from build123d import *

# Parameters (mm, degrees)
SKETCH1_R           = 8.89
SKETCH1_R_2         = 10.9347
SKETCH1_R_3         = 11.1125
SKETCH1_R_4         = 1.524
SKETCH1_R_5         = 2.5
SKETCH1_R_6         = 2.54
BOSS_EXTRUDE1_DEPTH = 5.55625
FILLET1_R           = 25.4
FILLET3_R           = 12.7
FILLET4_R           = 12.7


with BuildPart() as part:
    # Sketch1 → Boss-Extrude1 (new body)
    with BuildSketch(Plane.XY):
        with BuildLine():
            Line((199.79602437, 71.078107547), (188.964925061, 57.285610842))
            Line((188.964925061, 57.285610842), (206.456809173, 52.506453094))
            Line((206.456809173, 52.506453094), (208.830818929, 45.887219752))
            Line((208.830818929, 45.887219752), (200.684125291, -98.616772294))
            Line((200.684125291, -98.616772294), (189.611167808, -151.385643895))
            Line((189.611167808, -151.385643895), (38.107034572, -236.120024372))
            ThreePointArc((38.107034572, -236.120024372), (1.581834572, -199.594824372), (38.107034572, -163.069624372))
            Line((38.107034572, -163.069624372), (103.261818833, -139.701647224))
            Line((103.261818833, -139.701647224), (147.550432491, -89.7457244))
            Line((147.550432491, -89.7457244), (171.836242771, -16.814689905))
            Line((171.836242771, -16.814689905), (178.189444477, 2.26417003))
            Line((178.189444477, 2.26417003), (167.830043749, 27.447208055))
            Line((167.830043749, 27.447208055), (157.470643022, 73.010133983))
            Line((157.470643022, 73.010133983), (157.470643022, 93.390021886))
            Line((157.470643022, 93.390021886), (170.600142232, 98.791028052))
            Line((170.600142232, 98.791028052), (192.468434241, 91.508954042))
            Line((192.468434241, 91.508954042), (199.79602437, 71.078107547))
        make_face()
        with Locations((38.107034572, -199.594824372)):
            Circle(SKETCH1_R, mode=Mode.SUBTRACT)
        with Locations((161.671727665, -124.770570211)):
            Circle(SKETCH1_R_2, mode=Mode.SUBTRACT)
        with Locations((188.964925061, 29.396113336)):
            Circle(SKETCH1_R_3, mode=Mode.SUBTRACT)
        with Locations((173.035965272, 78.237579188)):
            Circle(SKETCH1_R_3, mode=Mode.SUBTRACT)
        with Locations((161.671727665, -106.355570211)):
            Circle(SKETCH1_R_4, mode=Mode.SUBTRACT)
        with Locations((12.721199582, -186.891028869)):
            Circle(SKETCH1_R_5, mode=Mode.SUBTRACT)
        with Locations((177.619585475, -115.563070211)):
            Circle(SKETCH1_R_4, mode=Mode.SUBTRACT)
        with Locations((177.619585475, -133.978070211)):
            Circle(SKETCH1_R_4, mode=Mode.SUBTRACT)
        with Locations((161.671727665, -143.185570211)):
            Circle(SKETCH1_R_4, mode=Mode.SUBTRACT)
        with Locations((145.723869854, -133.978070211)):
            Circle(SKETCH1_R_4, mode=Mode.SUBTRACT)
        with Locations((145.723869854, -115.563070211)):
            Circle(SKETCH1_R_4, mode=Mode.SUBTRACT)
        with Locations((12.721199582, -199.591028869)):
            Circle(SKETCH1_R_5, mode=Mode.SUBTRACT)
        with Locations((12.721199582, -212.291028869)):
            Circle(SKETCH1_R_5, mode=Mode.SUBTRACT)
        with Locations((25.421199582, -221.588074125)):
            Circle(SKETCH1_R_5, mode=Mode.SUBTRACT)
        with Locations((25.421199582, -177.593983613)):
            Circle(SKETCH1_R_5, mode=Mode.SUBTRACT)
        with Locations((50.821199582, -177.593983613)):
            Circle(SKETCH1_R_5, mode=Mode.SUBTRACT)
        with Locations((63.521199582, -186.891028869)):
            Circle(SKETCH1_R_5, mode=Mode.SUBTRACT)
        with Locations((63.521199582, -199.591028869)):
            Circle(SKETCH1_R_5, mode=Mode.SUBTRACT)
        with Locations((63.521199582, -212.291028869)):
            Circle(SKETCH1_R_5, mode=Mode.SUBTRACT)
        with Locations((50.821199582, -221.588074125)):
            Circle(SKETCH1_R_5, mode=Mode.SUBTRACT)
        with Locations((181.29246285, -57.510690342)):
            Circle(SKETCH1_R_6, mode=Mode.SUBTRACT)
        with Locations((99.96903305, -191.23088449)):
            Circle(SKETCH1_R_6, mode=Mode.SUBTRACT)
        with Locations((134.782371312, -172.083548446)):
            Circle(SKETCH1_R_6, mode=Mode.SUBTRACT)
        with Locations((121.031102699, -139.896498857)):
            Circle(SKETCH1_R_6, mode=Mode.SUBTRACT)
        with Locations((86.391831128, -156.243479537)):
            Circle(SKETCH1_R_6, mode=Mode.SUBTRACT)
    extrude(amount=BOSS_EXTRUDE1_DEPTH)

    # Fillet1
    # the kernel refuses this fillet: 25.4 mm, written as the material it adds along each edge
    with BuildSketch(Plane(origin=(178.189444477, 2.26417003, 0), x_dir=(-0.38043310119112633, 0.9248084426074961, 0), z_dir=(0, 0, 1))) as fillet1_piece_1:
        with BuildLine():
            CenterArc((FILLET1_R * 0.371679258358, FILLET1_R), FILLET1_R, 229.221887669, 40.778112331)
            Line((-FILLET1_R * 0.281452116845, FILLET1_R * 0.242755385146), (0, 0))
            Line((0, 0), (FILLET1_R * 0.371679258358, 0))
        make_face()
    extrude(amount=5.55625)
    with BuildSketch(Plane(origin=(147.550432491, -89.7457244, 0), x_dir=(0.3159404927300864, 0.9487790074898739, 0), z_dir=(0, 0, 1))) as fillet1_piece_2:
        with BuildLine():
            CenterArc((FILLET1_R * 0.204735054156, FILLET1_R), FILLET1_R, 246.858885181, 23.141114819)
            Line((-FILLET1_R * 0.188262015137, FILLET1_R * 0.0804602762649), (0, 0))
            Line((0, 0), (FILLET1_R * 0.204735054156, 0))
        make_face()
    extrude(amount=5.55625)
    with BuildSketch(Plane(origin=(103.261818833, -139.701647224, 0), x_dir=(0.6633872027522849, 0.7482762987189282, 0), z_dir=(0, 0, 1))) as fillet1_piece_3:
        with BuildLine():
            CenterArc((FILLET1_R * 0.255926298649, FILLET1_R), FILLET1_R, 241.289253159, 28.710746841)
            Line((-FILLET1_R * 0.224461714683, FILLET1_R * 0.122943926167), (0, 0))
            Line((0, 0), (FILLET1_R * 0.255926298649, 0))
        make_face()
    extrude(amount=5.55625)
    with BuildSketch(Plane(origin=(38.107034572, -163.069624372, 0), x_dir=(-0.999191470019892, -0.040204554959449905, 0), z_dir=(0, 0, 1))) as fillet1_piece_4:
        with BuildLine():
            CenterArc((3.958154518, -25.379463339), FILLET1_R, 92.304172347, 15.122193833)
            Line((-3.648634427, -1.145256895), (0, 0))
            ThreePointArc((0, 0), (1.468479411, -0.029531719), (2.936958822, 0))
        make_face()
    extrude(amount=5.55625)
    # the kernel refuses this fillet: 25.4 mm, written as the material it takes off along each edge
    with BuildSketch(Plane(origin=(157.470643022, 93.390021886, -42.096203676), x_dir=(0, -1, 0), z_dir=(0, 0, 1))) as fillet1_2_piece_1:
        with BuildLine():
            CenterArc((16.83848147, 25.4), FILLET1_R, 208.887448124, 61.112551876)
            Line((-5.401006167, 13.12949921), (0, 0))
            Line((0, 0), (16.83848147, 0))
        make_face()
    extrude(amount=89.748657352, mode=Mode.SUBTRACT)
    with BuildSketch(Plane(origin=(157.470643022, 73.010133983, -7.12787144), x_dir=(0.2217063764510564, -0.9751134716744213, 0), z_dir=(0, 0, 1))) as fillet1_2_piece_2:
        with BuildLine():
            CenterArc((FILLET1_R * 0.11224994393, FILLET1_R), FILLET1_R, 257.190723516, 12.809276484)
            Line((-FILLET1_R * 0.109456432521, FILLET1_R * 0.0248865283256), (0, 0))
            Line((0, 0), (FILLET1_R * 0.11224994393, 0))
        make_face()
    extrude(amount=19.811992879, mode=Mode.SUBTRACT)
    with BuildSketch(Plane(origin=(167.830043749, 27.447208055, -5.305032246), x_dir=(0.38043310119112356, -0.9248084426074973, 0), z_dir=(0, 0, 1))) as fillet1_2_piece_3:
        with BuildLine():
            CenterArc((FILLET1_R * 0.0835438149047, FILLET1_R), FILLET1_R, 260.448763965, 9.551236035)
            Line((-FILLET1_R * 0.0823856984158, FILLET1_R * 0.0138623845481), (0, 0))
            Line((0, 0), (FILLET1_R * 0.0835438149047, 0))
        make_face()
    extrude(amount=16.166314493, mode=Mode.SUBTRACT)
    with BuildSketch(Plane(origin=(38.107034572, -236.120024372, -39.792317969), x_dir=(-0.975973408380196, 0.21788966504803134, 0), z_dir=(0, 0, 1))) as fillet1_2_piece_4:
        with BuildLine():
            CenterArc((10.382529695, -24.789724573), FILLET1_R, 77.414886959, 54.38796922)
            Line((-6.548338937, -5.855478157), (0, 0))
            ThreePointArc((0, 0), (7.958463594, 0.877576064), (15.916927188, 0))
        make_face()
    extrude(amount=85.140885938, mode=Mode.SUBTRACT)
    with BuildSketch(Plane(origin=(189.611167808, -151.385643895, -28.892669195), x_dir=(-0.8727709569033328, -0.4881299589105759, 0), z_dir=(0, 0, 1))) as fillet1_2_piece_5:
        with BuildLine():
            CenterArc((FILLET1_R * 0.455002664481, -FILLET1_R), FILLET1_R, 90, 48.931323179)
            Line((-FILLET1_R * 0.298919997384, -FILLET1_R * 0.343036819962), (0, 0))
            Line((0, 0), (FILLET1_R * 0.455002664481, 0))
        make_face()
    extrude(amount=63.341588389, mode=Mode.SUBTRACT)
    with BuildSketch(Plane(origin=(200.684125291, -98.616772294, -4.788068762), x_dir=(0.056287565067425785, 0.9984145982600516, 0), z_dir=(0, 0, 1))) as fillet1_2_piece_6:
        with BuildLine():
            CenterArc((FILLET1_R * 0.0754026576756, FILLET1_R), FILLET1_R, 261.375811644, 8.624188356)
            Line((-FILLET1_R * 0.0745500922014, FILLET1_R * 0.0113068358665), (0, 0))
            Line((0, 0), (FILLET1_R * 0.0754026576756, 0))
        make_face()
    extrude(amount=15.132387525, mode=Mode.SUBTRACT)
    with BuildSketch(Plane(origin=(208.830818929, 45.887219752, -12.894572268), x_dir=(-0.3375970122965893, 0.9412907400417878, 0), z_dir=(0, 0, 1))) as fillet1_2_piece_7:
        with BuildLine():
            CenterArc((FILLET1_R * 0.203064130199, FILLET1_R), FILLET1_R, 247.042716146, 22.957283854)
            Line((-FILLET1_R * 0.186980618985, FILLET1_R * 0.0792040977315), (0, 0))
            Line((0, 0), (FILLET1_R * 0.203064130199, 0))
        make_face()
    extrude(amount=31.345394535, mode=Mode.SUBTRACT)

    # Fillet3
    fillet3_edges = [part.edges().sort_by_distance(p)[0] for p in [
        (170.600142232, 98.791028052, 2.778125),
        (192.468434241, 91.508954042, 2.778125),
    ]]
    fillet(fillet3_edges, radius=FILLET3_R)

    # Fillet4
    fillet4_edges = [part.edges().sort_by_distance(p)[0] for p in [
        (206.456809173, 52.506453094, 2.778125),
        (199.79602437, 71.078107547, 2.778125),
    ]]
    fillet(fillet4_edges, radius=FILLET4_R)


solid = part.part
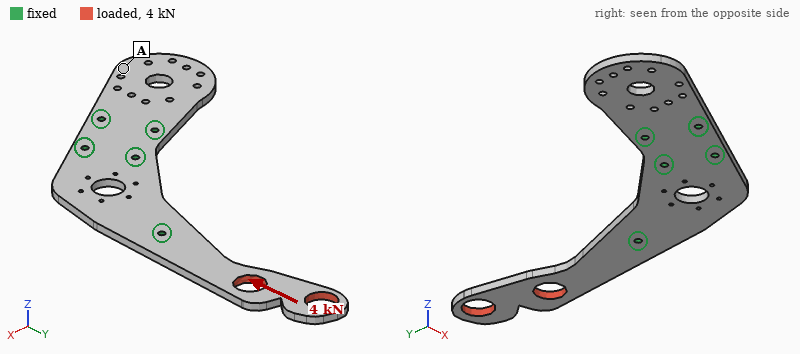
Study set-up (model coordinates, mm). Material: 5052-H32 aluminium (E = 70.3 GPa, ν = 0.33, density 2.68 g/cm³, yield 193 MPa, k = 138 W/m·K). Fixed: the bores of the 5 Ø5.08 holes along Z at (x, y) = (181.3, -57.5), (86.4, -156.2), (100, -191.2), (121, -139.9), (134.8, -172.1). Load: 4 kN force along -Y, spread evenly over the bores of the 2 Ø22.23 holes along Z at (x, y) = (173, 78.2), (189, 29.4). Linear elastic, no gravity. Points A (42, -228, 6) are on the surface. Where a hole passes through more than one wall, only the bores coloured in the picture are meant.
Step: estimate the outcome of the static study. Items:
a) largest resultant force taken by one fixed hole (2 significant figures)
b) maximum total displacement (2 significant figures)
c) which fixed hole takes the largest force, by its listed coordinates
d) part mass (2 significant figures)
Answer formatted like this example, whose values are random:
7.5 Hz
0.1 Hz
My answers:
3.6 kN
0.28 mm
(181.3, -57.5)
280 g
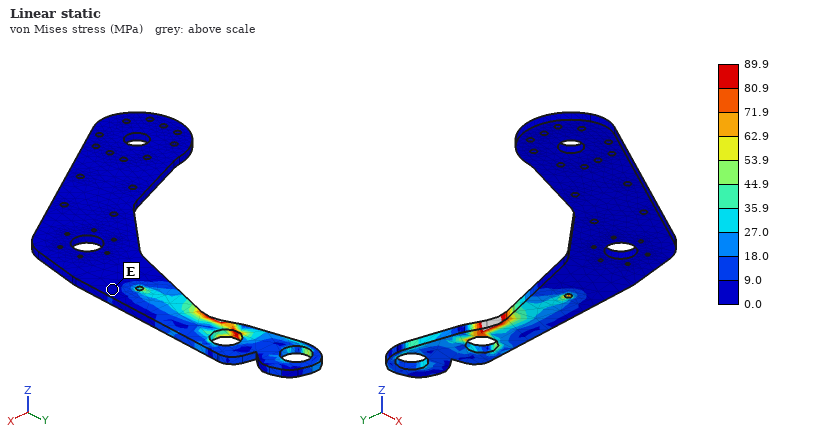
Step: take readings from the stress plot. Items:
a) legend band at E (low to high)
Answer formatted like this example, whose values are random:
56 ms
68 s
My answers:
0.0 to 9.0 MPa
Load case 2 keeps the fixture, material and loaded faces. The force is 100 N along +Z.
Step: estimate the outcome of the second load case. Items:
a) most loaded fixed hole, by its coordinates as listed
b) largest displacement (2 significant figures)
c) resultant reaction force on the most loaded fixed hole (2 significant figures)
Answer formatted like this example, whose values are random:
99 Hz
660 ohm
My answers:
(181.3, -57.5)
2.3 mm
120 N
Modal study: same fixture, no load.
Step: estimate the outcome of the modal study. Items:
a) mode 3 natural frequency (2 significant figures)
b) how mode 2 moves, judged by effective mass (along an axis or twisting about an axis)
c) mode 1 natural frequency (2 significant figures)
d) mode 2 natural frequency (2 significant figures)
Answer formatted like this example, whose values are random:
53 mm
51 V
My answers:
1100 Hz
along Z
220 Hz
530 Hz
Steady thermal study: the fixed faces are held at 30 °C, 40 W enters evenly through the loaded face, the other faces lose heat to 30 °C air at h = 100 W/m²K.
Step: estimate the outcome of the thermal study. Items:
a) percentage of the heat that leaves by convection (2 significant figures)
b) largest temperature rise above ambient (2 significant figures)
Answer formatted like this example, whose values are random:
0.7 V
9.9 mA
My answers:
83 %
60 K
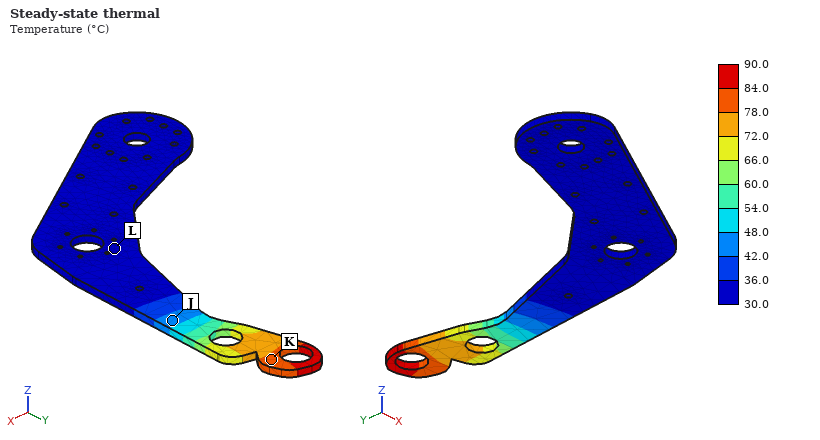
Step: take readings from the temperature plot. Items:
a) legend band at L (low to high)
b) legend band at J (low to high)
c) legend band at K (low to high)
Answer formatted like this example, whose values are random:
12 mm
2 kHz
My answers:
30.0 to 36.0 °C
42.0 to 48.0 °C
78.0 to 84.0 °C
